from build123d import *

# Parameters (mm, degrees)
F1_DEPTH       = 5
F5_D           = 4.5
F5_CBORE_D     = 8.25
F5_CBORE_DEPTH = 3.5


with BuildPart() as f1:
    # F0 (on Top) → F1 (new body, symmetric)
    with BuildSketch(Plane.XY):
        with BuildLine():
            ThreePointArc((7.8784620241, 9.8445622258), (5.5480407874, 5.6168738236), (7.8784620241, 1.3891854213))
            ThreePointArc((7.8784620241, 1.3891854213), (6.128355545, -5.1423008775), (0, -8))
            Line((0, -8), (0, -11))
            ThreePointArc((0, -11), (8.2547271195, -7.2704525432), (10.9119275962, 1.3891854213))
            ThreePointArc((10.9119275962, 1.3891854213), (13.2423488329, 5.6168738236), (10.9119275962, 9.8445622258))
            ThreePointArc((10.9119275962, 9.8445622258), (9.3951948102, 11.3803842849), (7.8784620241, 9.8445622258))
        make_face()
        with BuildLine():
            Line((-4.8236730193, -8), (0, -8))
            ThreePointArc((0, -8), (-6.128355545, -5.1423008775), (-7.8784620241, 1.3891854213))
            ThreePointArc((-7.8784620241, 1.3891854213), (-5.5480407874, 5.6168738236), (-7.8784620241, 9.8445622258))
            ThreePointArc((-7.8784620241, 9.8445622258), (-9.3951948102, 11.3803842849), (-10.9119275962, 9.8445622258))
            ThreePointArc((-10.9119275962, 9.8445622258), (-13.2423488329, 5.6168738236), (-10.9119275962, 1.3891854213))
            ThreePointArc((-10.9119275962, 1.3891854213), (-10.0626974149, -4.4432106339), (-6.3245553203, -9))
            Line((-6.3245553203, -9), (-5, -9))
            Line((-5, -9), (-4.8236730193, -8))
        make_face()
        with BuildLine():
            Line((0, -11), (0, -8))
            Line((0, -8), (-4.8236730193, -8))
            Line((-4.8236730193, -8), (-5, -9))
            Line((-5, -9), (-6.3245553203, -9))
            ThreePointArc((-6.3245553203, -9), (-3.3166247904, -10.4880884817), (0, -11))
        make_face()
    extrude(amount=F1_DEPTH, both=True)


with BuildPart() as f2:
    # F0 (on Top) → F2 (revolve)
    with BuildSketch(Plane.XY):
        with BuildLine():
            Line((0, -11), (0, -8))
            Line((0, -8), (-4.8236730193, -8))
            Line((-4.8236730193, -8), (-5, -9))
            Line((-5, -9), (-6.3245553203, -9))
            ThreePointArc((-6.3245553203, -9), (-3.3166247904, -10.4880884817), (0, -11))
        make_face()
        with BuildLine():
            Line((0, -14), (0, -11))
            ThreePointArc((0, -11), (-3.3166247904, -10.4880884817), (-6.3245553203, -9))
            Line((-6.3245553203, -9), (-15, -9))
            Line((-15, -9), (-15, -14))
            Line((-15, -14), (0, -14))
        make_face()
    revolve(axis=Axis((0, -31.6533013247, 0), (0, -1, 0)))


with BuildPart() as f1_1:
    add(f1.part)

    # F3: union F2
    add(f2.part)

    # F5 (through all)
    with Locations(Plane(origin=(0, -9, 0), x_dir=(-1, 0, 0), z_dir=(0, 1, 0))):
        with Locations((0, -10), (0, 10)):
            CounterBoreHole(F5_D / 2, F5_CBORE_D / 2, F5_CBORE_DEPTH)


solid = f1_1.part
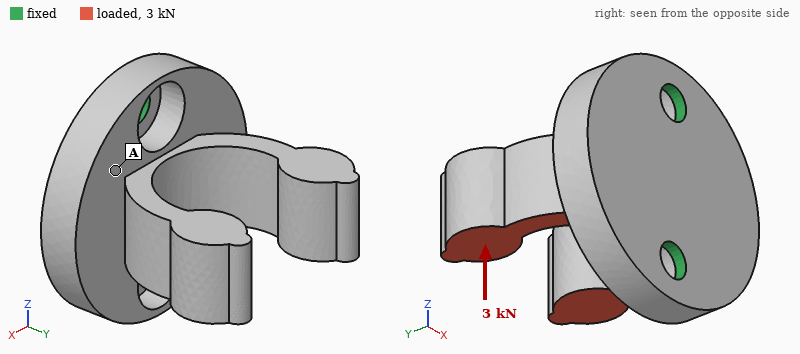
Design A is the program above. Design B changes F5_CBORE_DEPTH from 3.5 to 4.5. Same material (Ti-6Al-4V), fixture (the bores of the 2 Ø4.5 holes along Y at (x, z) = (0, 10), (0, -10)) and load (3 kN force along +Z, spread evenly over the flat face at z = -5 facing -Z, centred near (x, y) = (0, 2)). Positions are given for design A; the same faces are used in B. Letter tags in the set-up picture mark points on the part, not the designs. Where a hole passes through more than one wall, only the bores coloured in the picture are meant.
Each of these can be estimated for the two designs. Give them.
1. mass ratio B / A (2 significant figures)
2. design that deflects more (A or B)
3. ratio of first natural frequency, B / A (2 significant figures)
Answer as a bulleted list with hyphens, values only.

- 0.99
- B
- 0.49
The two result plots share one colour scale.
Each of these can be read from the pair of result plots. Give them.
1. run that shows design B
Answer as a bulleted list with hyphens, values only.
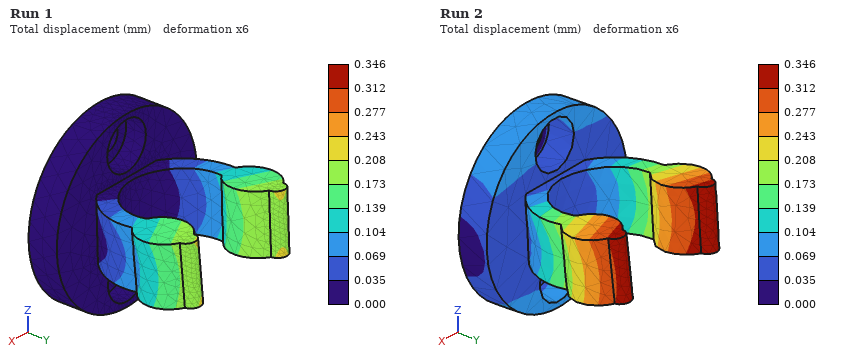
- Run 2
